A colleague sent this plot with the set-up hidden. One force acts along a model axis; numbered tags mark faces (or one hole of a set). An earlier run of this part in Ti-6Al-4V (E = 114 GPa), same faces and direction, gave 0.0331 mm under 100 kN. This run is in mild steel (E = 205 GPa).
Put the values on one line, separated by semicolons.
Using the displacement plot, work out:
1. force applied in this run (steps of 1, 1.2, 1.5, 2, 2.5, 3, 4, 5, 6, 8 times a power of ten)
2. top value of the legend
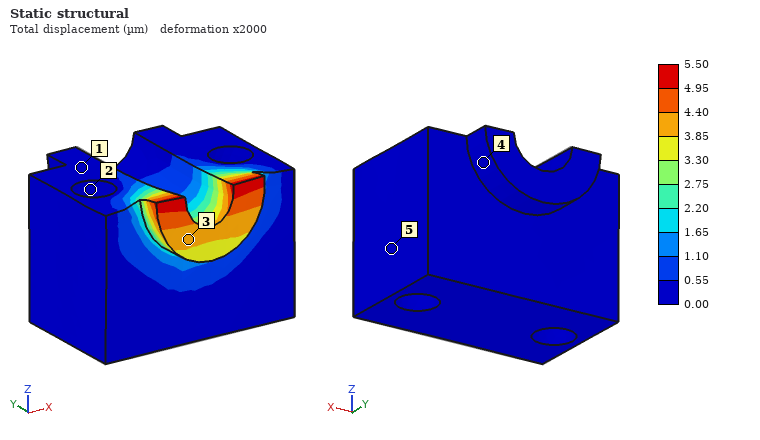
30 kN; 5.50 µm
